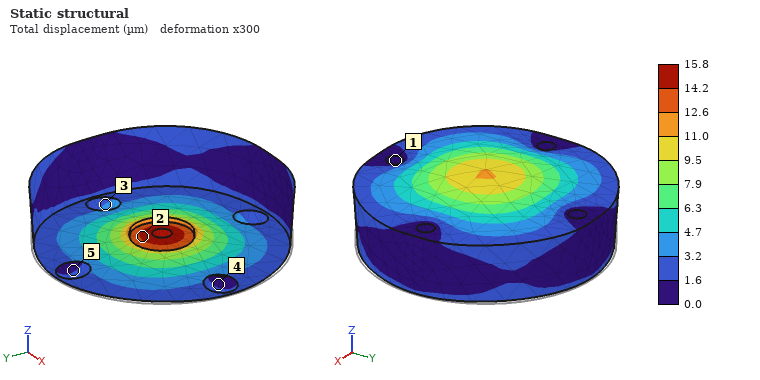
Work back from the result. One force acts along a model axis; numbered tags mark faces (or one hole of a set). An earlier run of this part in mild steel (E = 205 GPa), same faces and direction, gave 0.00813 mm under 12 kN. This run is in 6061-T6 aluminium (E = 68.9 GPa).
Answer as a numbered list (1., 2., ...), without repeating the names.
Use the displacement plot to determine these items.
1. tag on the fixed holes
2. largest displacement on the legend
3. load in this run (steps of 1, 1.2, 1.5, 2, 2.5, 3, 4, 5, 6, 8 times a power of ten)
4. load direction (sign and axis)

1. 1
2. 15.8 µm
3. 8 kN
4. +Z
